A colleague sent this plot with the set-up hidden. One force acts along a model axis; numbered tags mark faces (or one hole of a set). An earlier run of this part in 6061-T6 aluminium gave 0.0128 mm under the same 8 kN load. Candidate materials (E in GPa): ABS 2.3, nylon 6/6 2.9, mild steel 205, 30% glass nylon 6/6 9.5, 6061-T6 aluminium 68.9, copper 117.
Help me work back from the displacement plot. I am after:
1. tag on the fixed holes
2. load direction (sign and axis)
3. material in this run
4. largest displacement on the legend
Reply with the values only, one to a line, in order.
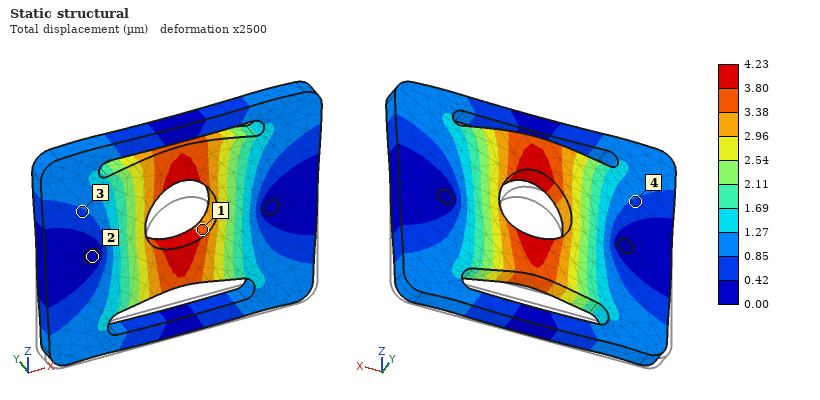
2
+Z
mild steel
4.23 µm
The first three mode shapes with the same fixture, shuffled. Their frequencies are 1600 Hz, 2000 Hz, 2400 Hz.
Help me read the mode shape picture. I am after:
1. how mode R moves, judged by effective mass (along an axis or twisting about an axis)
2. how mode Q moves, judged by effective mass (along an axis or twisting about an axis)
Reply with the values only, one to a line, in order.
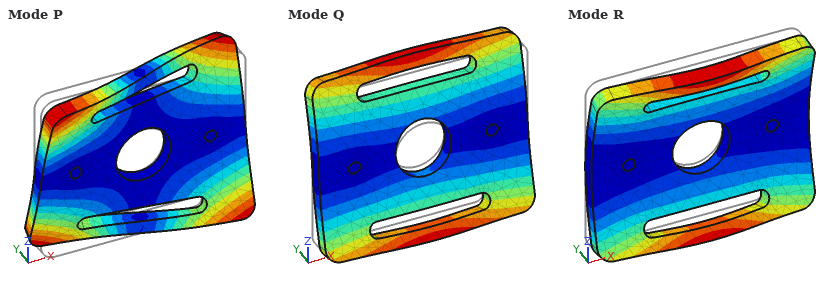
along Y
twisting about X
